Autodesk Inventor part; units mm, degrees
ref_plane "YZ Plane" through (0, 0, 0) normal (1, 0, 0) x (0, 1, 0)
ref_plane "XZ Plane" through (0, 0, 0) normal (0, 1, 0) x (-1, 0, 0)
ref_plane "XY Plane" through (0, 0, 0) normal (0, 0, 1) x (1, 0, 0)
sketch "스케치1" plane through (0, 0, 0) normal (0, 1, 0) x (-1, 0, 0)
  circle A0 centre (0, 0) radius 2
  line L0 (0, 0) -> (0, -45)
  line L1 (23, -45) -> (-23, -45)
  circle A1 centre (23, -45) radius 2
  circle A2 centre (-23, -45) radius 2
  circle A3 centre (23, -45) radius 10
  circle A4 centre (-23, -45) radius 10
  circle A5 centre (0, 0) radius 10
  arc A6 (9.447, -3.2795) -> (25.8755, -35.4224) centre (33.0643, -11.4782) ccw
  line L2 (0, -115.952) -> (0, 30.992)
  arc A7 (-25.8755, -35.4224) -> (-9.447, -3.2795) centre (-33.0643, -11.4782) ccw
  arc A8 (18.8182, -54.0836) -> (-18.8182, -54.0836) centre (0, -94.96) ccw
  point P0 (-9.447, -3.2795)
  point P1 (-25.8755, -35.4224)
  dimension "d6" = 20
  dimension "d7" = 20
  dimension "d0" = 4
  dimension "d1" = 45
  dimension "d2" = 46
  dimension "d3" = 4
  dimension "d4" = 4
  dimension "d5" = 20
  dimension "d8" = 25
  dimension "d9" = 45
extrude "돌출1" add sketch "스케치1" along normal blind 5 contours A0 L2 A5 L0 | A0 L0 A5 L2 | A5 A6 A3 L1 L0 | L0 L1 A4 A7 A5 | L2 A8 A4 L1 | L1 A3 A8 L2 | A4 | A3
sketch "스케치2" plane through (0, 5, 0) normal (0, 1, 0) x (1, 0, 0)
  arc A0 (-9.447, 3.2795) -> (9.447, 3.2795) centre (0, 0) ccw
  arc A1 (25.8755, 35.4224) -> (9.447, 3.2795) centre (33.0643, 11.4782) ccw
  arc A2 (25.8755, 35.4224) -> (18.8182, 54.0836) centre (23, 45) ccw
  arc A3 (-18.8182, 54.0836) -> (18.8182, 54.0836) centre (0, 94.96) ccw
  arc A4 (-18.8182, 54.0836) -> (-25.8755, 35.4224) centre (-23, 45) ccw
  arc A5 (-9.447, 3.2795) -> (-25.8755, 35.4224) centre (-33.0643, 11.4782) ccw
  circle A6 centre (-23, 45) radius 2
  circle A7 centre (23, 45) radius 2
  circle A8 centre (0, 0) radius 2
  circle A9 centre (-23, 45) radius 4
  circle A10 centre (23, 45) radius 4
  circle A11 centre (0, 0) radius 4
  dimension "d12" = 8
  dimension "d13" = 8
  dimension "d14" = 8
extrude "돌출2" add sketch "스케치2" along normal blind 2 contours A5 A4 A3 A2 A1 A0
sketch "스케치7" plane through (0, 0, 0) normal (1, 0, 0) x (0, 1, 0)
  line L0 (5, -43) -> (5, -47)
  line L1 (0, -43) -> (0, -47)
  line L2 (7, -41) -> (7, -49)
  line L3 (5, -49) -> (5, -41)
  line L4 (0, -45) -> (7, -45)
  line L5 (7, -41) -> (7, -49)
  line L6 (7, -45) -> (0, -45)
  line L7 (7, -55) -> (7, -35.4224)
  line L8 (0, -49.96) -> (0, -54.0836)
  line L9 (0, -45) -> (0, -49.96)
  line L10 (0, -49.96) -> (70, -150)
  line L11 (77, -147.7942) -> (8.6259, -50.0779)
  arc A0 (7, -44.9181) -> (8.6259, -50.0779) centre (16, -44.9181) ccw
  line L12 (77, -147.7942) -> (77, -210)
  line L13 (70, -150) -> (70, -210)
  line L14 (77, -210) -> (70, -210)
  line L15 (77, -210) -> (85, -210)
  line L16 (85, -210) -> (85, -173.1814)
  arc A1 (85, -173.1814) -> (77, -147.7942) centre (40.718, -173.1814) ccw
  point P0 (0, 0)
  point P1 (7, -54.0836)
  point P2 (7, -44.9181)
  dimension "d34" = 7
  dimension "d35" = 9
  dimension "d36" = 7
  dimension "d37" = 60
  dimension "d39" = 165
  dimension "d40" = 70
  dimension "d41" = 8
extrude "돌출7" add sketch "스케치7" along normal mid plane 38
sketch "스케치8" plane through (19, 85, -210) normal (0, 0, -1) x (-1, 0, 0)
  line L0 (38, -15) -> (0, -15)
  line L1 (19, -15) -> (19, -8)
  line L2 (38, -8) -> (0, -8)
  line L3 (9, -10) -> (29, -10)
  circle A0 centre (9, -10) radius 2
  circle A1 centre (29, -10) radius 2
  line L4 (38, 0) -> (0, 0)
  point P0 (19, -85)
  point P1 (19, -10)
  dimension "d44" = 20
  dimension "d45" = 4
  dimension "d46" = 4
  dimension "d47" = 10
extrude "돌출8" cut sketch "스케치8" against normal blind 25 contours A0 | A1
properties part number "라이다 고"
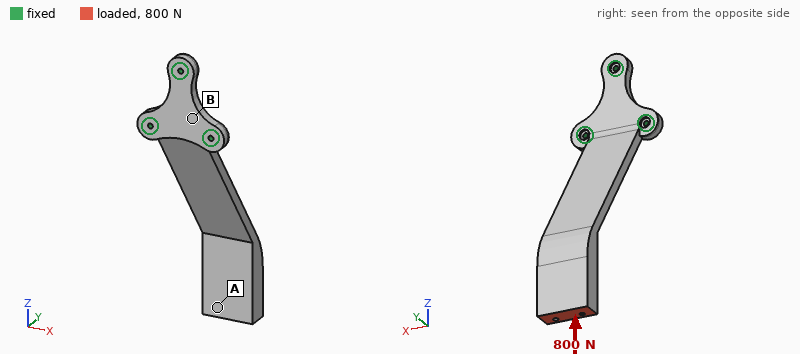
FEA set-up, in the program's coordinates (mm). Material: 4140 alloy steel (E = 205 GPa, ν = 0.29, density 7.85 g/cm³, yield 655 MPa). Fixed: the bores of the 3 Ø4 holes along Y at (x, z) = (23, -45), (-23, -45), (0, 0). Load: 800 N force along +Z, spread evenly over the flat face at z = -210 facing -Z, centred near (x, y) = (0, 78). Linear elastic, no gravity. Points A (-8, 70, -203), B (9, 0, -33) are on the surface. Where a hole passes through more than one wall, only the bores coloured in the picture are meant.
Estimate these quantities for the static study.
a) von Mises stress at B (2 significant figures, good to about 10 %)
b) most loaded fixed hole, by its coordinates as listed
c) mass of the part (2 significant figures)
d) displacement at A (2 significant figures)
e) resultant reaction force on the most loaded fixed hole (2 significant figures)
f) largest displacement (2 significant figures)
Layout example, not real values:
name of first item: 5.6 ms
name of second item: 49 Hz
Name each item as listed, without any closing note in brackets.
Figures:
von Mises stress at B: 42 MPa
most loaded fixed hole, by its coordinates as listed: (0, 0)
mass of the part: 610 g
displacement at A: 2.5 mm
resultant reaction force on the most loaded fixed hole: 1.6 kN
largest displacement: 2.7 mm
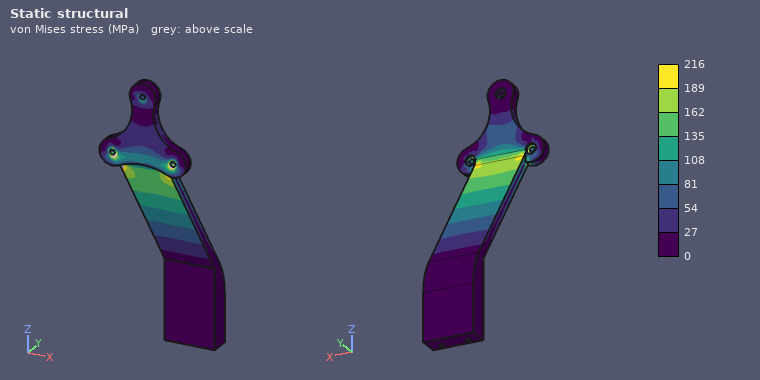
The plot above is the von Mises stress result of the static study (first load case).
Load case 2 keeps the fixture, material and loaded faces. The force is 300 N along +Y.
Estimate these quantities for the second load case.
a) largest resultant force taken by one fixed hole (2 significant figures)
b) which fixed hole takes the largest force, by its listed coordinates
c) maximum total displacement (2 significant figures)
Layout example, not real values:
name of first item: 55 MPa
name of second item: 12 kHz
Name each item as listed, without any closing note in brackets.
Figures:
largest resultant force taken by one fixed hole: 1.2 kN
which fixed hole takes the largest force, by its listed coordinates: (0, 0)
maximum total displacement: 2.7 mm
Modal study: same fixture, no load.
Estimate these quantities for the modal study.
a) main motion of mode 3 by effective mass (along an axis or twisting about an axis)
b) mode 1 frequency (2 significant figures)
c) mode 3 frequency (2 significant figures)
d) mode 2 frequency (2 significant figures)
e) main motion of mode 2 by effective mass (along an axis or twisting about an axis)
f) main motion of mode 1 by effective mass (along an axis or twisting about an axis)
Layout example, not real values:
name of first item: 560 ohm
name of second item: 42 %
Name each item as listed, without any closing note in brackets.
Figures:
main motion of mode 3 by effective mass: along Z
mode 1 frequency: 120 Hz
mode 3 frequency: 880 Hz
mode 2 frequency: 540 Hz
main motion of mode 2 by effective mass: along X
main motion of mode 1 by effective mass: along Y
